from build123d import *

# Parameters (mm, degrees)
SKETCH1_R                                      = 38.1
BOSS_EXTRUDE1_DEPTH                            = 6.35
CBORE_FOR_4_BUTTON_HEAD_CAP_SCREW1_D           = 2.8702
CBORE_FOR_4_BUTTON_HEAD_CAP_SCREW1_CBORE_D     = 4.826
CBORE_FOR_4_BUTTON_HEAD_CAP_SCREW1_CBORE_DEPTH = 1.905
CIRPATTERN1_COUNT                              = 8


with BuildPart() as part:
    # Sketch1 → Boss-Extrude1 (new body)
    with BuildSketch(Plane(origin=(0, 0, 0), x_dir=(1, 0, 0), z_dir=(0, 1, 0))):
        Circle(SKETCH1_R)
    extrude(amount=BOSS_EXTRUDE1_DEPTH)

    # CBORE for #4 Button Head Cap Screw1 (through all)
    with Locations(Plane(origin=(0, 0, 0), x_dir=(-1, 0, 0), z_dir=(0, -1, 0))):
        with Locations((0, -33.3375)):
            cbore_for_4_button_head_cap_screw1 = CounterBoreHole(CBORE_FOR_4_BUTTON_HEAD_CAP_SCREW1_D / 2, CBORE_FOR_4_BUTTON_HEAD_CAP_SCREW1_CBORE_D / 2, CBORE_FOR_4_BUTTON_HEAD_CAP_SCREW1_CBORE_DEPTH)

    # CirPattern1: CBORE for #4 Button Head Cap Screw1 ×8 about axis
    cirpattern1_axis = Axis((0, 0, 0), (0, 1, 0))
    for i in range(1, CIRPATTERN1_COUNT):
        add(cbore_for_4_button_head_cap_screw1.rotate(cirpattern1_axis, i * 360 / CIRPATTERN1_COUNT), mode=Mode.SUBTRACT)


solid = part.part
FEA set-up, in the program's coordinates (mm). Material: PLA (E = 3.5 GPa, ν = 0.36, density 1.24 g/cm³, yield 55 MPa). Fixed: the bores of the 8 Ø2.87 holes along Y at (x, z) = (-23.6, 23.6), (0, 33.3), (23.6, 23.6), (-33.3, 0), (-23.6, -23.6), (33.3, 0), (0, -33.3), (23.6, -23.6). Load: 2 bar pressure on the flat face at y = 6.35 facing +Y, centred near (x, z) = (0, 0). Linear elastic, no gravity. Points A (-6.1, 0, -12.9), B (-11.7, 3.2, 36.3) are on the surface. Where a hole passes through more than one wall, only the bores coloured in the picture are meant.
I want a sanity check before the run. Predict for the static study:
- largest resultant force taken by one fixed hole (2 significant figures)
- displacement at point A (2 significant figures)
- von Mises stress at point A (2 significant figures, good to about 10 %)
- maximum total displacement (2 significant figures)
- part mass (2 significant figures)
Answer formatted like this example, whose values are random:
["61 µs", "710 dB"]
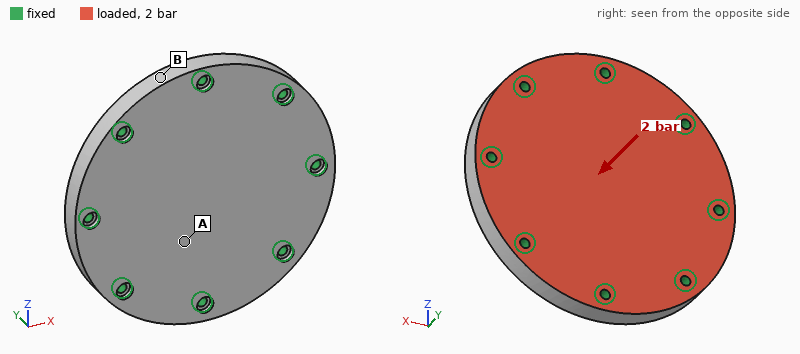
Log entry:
["120 N", "69 µm", "3.1 MPa", "90 µm", "35 g"]
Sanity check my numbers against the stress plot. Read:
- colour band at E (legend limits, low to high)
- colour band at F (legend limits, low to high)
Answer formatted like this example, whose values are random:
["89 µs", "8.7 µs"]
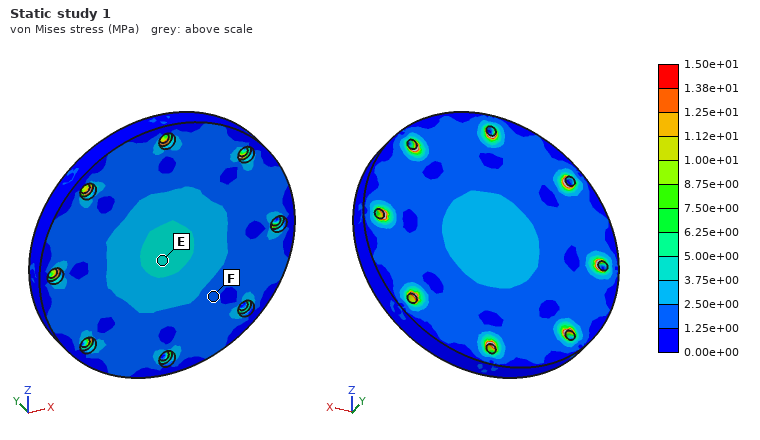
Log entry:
["3.75e+00 to 5.00e+00 MPa", "1.25e+00 to 2.50e+00 MPa"]
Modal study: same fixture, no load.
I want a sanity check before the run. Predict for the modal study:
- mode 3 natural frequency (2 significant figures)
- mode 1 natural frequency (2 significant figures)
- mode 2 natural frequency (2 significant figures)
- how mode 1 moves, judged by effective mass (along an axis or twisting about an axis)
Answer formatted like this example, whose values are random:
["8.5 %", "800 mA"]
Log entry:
["6700 Hz", "3200 Hz", "6700 Hz", "along Y"]
